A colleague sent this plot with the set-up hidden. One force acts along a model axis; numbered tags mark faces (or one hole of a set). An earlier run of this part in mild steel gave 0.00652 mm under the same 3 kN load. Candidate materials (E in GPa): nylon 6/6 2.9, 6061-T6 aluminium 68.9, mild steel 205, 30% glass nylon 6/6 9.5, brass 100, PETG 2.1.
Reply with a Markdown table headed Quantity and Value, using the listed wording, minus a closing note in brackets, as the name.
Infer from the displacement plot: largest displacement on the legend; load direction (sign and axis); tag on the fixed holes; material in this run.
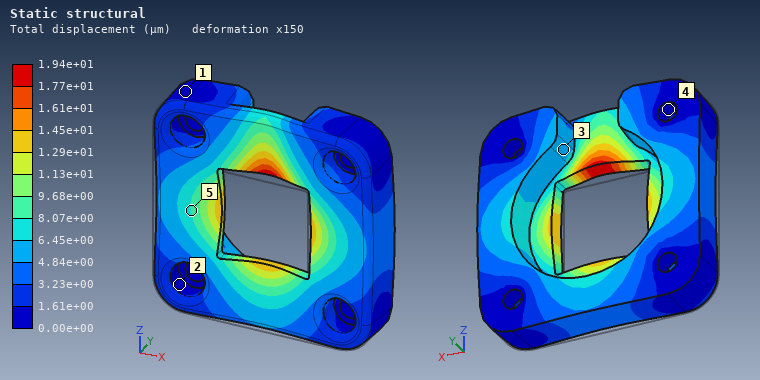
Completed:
| Quantity | Value |
|---|---|
| largest displacement on the legend | 1.94e+01 µm |
| load direction | +Y |
| tag on the fixed holes | 4 |
| material in this run | 6061-T6 aluminium |
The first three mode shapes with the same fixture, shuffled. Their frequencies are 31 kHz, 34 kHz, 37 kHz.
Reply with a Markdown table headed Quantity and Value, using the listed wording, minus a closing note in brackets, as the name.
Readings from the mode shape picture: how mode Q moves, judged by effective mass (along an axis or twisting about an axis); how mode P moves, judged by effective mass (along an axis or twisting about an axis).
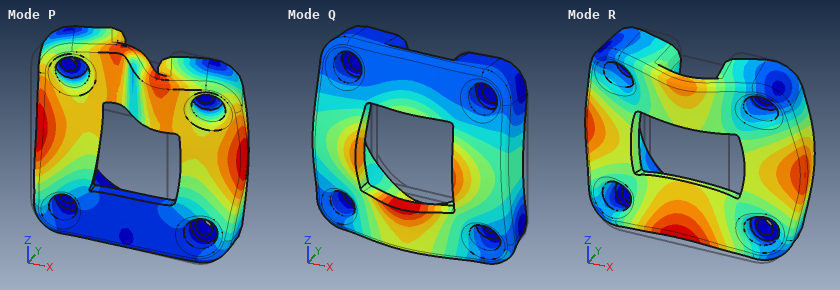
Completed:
| Quantity | Value |
|---|---|
| how mode Q moves, judged by effective mass | along Y |
| how mode P moves, judged by effective mass | along X |
